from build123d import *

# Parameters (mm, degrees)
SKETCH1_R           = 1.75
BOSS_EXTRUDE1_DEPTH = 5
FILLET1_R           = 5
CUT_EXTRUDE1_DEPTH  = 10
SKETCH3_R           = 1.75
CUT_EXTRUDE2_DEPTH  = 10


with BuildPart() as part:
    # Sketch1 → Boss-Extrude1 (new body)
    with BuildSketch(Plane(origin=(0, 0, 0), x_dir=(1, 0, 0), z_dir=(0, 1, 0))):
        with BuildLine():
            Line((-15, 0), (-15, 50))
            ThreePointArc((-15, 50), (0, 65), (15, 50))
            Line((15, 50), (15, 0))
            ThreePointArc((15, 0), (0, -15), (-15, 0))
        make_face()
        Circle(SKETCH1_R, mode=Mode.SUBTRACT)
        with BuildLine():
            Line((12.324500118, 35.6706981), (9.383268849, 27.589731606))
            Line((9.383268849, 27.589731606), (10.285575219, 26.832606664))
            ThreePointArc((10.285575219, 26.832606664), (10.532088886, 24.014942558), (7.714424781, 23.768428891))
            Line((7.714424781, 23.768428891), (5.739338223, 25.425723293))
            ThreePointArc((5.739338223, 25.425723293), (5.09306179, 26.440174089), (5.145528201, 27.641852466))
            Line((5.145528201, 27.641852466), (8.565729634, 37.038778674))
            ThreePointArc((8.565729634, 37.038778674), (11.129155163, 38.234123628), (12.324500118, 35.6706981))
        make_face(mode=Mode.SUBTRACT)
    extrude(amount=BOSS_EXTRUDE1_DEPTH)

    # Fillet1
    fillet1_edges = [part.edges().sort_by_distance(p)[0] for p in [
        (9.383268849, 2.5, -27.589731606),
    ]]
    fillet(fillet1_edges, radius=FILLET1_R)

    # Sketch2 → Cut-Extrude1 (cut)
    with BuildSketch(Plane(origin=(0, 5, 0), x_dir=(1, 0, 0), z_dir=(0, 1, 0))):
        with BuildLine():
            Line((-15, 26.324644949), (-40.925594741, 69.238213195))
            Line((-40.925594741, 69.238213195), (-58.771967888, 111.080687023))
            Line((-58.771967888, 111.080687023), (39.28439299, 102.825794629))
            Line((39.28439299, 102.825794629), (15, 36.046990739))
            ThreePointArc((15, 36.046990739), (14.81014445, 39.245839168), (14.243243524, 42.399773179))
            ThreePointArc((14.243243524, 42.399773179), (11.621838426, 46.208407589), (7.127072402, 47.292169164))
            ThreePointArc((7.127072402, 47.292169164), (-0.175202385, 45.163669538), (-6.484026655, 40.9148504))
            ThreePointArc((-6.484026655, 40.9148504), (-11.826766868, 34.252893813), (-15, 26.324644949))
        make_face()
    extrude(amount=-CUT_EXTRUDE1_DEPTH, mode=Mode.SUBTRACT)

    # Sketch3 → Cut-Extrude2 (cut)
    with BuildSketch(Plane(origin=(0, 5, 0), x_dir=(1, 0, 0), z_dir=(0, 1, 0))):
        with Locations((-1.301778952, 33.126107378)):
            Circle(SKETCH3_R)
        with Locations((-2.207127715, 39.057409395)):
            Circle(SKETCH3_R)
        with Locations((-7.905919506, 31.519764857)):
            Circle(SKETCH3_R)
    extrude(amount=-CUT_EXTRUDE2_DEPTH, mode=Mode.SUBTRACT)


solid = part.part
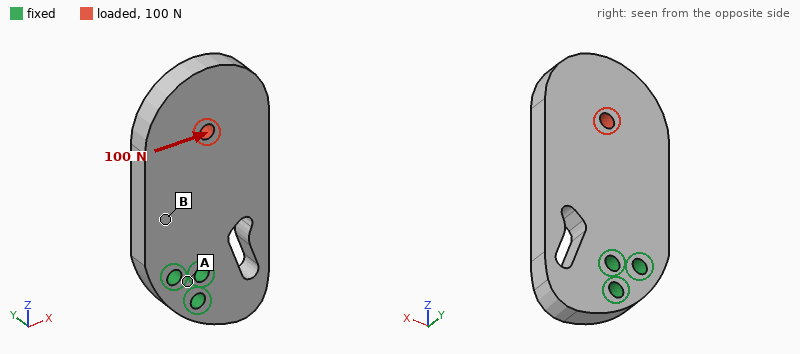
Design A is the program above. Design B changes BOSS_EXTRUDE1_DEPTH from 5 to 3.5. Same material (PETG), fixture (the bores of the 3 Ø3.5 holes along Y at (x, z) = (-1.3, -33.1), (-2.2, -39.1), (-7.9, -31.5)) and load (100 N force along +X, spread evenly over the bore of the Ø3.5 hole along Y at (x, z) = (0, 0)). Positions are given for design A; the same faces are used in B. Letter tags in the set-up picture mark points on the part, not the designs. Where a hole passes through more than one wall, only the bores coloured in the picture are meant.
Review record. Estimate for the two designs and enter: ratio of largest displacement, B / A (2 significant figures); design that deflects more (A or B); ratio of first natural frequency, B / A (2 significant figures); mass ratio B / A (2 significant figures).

1.4
B
0.72
0.70
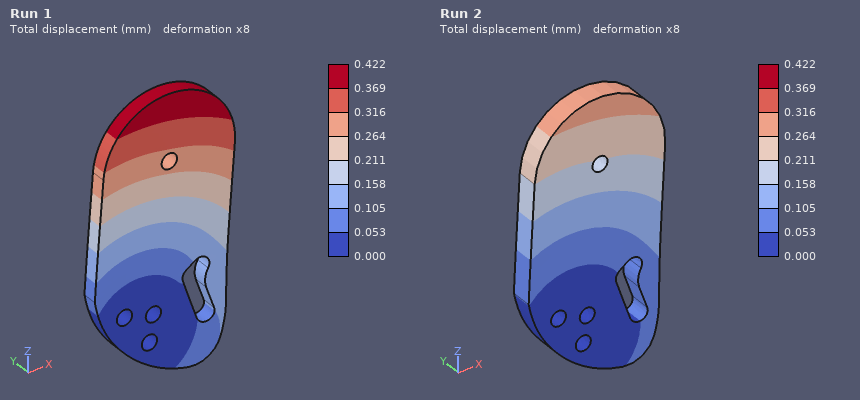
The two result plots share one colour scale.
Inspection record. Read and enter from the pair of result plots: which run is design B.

Run 1
